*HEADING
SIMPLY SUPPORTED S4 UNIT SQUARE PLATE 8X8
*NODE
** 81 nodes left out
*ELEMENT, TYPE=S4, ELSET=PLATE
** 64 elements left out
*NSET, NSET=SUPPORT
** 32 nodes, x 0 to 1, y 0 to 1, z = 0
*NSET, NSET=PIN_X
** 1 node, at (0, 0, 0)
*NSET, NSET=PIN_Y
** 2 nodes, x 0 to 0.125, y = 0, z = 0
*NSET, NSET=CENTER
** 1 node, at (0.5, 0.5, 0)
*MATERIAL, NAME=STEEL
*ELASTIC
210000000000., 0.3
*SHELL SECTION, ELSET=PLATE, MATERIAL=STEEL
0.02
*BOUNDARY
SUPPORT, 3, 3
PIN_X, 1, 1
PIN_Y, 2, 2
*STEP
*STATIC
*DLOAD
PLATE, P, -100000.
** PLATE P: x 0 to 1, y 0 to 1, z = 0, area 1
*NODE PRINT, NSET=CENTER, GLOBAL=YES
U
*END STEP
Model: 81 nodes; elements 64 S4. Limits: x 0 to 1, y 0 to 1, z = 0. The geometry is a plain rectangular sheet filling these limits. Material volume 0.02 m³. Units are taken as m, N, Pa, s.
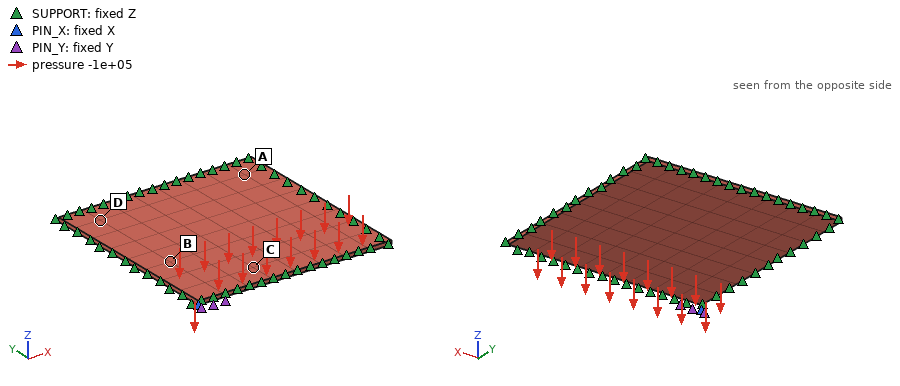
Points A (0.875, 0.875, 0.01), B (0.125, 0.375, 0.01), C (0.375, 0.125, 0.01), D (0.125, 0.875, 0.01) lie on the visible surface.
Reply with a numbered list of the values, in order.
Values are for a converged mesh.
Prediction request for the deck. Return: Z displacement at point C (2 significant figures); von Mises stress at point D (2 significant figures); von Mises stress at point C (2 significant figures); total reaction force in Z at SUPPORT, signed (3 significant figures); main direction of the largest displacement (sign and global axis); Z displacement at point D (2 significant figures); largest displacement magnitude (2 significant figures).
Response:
1. -0.0010 m
2. 7.3e+07 Pa
3. 4.3e+07 Pa
4. 1.00e+05 N
5. -Z
6. -4.4e-04 m
7. 0.0027 m
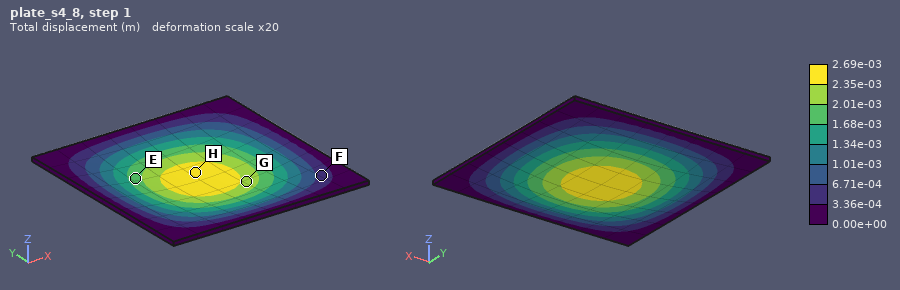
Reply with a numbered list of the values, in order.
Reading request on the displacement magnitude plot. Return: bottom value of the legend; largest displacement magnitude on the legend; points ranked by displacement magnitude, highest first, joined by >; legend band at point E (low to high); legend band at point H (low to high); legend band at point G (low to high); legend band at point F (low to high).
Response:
1. 0.00e+00 m
2. 2.69e-03 m
3. H > G > E > F
4. 1.68e-03 to 2.01e-03 m
5. 2.35e-03 to 2.69e-03 m
6. 2.01e-03 to 2.35e-03 m
7. 3.36e-04 to 6.71e-04 m
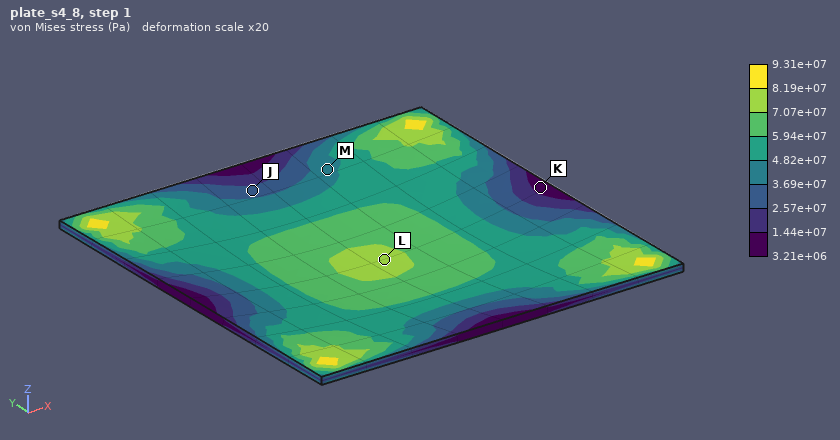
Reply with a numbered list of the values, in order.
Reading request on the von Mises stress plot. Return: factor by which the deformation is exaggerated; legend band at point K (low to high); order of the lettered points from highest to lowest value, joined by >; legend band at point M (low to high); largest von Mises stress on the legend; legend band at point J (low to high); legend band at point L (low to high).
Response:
1. 20
2. 3.21e+06 to 1.44e+07 Pa
3. L > M > J > K
4. 3.69e+07 to 4.82e+07 Pa
5. 9.31e+07 Pa
6. 2.57e+07 to 3.69e+07 Pa
7. 7.07e+07 to 8.19e+07 Pa
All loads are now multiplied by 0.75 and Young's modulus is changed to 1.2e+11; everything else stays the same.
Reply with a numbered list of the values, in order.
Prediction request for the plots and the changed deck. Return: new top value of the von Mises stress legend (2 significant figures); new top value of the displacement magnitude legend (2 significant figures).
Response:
1. 7.0e+07 Pa
2. 0.0035 m
